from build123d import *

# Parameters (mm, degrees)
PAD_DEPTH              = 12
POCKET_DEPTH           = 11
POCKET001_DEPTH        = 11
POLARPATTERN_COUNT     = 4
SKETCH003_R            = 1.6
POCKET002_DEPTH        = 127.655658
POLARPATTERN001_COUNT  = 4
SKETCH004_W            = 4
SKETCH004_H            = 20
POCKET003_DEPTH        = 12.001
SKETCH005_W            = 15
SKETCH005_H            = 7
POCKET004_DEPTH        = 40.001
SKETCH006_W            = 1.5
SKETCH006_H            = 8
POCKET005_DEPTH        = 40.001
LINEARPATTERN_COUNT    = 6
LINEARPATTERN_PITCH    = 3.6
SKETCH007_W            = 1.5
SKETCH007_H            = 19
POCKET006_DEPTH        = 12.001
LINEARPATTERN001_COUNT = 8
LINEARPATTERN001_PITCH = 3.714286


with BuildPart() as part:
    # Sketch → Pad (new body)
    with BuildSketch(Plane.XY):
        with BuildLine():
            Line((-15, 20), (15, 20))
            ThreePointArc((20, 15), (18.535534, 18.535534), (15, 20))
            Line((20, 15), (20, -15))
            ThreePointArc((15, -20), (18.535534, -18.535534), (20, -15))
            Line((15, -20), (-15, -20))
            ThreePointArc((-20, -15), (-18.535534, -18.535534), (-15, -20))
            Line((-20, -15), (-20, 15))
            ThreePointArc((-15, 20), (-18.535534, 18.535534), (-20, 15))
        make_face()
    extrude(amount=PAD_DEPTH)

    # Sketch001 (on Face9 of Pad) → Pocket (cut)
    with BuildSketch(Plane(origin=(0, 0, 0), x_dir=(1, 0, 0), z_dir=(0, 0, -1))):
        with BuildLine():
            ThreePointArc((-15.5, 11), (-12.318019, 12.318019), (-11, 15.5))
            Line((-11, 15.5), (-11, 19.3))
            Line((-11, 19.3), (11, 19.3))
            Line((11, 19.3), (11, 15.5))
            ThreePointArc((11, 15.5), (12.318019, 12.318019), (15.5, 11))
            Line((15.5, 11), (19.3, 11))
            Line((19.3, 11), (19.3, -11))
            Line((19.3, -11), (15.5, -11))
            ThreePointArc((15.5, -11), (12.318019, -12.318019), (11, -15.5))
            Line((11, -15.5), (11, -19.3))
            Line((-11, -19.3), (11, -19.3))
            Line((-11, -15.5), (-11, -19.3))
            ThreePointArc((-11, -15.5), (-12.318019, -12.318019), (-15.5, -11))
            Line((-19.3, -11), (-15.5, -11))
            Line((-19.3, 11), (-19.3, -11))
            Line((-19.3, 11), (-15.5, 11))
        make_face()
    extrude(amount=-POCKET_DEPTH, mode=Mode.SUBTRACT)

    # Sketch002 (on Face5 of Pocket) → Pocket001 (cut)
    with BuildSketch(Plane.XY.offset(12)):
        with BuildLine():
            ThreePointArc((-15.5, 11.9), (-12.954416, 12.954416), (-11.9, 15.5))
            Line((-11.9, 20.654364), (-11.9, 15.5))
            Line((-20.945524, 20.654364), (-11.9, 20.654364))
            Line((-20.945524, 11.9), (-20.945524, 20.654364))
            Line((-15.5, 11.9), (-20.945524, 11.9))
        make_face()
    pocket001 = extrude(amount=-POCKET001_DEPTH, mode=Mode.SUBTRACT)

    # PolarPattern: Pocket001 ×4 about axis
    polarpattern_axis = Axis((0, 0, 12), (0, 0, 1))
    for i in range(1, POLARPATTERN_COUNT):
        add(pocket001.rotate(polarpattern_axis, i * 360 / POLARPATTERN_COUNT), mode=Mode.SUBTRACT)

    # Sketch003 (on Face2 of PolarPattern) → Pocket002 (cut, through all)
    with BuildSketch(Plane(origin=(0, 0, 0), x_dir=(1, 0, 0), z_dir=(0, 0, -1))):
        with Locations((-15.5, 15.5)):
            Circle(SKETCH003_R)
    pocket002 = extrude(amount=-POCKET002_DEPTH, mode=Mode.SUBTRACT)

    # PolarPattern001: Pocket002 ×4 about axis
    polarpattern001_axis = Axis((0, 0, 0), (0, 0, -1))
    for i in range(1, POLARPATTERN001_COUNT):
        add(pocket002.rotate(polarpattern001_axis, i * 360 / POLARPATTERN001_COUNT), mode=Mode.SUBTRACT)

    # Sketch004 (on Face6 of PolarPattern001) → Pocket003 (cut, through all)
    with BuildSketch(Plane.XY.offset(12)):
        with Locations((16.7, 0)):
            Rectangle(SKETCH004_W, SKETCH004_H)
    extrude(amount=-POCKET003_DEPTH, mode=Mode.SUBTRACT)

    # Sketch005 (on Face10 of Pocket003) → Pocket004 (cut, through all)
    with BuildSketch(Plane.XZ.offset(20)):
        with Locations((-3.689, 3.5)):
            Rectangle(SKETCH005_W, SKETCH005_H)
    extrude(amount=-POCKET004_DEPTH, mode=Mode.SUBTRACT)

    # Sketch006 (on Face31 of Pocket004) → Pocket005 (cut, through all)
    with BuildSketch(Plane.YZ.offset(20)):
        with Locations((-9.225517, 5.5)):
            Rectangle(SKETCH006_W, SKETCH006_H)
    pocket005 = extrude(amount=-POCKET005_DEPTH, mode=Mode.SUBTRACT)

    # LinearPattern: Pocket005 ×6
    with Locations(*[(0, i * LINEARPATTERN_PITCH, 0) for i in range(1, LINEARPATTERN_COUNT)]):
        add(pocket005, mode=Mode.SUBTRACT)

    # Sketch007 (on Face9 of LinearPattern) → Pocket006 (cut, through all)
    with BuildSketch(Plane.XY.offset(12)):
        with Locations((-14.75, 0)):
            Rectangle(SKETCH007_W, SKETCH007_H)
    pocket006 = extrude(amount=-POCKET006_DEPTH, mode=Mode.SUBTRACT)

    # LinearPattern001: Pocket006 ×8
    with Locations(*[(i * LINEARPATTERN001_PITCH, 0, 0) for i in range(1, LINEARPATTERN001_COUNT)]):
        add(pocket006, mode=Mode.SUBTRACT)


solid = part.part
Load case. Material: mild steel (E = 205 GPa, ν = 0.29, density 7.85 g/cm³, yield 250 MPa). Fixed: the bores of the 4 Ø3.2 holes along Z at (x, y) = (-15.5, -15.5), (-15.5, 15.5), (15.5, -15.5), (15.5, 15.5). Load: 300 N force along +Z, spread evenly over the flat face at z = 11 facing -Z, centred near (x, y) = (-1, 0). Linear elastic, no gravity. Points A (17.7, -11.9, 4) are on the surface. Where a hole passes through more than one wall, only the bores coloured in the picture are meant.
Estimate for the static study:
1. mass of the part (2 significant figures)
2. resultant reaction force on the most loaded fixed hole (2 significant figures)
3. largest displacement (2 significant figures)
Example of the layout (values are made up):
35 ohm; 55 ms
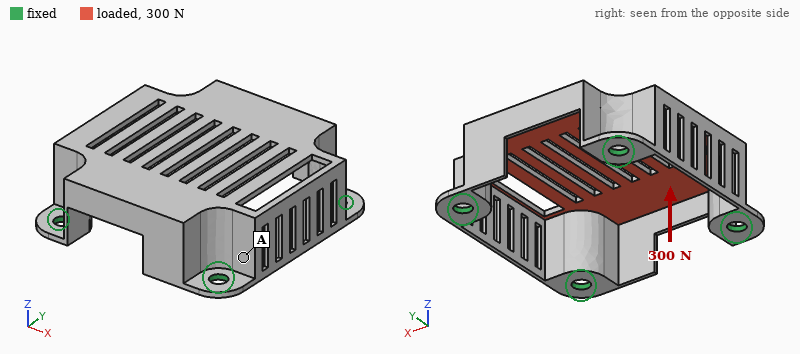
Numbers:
18 g; 85 N; 75 µm
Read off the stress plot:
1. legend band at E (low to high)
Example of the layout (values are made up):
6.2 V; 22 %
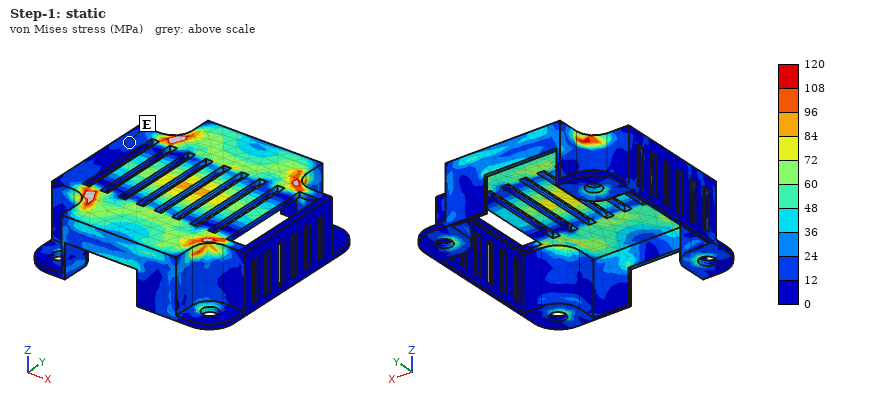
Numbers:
12 to 24 MPa
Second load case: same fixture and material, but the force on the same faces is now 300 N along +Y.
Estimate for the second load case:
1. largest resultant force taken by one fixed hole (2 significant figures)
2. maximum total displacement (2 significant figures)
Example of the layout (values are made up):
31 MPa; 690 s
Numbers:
100 N; 15 µm
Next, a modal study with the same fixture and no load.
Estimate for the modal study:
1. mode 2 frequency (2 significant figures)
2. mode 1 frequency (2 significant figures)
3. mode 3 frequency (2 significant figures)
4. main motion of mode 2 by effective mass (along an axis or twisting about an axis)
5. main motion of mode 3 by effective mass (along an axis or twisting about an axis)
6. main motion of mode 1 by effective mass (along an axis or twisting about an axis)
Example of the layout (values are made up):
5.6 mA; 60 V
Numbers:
6300 Hz; 4900 Hz; 7100 Hz; along X; along X; along Z
